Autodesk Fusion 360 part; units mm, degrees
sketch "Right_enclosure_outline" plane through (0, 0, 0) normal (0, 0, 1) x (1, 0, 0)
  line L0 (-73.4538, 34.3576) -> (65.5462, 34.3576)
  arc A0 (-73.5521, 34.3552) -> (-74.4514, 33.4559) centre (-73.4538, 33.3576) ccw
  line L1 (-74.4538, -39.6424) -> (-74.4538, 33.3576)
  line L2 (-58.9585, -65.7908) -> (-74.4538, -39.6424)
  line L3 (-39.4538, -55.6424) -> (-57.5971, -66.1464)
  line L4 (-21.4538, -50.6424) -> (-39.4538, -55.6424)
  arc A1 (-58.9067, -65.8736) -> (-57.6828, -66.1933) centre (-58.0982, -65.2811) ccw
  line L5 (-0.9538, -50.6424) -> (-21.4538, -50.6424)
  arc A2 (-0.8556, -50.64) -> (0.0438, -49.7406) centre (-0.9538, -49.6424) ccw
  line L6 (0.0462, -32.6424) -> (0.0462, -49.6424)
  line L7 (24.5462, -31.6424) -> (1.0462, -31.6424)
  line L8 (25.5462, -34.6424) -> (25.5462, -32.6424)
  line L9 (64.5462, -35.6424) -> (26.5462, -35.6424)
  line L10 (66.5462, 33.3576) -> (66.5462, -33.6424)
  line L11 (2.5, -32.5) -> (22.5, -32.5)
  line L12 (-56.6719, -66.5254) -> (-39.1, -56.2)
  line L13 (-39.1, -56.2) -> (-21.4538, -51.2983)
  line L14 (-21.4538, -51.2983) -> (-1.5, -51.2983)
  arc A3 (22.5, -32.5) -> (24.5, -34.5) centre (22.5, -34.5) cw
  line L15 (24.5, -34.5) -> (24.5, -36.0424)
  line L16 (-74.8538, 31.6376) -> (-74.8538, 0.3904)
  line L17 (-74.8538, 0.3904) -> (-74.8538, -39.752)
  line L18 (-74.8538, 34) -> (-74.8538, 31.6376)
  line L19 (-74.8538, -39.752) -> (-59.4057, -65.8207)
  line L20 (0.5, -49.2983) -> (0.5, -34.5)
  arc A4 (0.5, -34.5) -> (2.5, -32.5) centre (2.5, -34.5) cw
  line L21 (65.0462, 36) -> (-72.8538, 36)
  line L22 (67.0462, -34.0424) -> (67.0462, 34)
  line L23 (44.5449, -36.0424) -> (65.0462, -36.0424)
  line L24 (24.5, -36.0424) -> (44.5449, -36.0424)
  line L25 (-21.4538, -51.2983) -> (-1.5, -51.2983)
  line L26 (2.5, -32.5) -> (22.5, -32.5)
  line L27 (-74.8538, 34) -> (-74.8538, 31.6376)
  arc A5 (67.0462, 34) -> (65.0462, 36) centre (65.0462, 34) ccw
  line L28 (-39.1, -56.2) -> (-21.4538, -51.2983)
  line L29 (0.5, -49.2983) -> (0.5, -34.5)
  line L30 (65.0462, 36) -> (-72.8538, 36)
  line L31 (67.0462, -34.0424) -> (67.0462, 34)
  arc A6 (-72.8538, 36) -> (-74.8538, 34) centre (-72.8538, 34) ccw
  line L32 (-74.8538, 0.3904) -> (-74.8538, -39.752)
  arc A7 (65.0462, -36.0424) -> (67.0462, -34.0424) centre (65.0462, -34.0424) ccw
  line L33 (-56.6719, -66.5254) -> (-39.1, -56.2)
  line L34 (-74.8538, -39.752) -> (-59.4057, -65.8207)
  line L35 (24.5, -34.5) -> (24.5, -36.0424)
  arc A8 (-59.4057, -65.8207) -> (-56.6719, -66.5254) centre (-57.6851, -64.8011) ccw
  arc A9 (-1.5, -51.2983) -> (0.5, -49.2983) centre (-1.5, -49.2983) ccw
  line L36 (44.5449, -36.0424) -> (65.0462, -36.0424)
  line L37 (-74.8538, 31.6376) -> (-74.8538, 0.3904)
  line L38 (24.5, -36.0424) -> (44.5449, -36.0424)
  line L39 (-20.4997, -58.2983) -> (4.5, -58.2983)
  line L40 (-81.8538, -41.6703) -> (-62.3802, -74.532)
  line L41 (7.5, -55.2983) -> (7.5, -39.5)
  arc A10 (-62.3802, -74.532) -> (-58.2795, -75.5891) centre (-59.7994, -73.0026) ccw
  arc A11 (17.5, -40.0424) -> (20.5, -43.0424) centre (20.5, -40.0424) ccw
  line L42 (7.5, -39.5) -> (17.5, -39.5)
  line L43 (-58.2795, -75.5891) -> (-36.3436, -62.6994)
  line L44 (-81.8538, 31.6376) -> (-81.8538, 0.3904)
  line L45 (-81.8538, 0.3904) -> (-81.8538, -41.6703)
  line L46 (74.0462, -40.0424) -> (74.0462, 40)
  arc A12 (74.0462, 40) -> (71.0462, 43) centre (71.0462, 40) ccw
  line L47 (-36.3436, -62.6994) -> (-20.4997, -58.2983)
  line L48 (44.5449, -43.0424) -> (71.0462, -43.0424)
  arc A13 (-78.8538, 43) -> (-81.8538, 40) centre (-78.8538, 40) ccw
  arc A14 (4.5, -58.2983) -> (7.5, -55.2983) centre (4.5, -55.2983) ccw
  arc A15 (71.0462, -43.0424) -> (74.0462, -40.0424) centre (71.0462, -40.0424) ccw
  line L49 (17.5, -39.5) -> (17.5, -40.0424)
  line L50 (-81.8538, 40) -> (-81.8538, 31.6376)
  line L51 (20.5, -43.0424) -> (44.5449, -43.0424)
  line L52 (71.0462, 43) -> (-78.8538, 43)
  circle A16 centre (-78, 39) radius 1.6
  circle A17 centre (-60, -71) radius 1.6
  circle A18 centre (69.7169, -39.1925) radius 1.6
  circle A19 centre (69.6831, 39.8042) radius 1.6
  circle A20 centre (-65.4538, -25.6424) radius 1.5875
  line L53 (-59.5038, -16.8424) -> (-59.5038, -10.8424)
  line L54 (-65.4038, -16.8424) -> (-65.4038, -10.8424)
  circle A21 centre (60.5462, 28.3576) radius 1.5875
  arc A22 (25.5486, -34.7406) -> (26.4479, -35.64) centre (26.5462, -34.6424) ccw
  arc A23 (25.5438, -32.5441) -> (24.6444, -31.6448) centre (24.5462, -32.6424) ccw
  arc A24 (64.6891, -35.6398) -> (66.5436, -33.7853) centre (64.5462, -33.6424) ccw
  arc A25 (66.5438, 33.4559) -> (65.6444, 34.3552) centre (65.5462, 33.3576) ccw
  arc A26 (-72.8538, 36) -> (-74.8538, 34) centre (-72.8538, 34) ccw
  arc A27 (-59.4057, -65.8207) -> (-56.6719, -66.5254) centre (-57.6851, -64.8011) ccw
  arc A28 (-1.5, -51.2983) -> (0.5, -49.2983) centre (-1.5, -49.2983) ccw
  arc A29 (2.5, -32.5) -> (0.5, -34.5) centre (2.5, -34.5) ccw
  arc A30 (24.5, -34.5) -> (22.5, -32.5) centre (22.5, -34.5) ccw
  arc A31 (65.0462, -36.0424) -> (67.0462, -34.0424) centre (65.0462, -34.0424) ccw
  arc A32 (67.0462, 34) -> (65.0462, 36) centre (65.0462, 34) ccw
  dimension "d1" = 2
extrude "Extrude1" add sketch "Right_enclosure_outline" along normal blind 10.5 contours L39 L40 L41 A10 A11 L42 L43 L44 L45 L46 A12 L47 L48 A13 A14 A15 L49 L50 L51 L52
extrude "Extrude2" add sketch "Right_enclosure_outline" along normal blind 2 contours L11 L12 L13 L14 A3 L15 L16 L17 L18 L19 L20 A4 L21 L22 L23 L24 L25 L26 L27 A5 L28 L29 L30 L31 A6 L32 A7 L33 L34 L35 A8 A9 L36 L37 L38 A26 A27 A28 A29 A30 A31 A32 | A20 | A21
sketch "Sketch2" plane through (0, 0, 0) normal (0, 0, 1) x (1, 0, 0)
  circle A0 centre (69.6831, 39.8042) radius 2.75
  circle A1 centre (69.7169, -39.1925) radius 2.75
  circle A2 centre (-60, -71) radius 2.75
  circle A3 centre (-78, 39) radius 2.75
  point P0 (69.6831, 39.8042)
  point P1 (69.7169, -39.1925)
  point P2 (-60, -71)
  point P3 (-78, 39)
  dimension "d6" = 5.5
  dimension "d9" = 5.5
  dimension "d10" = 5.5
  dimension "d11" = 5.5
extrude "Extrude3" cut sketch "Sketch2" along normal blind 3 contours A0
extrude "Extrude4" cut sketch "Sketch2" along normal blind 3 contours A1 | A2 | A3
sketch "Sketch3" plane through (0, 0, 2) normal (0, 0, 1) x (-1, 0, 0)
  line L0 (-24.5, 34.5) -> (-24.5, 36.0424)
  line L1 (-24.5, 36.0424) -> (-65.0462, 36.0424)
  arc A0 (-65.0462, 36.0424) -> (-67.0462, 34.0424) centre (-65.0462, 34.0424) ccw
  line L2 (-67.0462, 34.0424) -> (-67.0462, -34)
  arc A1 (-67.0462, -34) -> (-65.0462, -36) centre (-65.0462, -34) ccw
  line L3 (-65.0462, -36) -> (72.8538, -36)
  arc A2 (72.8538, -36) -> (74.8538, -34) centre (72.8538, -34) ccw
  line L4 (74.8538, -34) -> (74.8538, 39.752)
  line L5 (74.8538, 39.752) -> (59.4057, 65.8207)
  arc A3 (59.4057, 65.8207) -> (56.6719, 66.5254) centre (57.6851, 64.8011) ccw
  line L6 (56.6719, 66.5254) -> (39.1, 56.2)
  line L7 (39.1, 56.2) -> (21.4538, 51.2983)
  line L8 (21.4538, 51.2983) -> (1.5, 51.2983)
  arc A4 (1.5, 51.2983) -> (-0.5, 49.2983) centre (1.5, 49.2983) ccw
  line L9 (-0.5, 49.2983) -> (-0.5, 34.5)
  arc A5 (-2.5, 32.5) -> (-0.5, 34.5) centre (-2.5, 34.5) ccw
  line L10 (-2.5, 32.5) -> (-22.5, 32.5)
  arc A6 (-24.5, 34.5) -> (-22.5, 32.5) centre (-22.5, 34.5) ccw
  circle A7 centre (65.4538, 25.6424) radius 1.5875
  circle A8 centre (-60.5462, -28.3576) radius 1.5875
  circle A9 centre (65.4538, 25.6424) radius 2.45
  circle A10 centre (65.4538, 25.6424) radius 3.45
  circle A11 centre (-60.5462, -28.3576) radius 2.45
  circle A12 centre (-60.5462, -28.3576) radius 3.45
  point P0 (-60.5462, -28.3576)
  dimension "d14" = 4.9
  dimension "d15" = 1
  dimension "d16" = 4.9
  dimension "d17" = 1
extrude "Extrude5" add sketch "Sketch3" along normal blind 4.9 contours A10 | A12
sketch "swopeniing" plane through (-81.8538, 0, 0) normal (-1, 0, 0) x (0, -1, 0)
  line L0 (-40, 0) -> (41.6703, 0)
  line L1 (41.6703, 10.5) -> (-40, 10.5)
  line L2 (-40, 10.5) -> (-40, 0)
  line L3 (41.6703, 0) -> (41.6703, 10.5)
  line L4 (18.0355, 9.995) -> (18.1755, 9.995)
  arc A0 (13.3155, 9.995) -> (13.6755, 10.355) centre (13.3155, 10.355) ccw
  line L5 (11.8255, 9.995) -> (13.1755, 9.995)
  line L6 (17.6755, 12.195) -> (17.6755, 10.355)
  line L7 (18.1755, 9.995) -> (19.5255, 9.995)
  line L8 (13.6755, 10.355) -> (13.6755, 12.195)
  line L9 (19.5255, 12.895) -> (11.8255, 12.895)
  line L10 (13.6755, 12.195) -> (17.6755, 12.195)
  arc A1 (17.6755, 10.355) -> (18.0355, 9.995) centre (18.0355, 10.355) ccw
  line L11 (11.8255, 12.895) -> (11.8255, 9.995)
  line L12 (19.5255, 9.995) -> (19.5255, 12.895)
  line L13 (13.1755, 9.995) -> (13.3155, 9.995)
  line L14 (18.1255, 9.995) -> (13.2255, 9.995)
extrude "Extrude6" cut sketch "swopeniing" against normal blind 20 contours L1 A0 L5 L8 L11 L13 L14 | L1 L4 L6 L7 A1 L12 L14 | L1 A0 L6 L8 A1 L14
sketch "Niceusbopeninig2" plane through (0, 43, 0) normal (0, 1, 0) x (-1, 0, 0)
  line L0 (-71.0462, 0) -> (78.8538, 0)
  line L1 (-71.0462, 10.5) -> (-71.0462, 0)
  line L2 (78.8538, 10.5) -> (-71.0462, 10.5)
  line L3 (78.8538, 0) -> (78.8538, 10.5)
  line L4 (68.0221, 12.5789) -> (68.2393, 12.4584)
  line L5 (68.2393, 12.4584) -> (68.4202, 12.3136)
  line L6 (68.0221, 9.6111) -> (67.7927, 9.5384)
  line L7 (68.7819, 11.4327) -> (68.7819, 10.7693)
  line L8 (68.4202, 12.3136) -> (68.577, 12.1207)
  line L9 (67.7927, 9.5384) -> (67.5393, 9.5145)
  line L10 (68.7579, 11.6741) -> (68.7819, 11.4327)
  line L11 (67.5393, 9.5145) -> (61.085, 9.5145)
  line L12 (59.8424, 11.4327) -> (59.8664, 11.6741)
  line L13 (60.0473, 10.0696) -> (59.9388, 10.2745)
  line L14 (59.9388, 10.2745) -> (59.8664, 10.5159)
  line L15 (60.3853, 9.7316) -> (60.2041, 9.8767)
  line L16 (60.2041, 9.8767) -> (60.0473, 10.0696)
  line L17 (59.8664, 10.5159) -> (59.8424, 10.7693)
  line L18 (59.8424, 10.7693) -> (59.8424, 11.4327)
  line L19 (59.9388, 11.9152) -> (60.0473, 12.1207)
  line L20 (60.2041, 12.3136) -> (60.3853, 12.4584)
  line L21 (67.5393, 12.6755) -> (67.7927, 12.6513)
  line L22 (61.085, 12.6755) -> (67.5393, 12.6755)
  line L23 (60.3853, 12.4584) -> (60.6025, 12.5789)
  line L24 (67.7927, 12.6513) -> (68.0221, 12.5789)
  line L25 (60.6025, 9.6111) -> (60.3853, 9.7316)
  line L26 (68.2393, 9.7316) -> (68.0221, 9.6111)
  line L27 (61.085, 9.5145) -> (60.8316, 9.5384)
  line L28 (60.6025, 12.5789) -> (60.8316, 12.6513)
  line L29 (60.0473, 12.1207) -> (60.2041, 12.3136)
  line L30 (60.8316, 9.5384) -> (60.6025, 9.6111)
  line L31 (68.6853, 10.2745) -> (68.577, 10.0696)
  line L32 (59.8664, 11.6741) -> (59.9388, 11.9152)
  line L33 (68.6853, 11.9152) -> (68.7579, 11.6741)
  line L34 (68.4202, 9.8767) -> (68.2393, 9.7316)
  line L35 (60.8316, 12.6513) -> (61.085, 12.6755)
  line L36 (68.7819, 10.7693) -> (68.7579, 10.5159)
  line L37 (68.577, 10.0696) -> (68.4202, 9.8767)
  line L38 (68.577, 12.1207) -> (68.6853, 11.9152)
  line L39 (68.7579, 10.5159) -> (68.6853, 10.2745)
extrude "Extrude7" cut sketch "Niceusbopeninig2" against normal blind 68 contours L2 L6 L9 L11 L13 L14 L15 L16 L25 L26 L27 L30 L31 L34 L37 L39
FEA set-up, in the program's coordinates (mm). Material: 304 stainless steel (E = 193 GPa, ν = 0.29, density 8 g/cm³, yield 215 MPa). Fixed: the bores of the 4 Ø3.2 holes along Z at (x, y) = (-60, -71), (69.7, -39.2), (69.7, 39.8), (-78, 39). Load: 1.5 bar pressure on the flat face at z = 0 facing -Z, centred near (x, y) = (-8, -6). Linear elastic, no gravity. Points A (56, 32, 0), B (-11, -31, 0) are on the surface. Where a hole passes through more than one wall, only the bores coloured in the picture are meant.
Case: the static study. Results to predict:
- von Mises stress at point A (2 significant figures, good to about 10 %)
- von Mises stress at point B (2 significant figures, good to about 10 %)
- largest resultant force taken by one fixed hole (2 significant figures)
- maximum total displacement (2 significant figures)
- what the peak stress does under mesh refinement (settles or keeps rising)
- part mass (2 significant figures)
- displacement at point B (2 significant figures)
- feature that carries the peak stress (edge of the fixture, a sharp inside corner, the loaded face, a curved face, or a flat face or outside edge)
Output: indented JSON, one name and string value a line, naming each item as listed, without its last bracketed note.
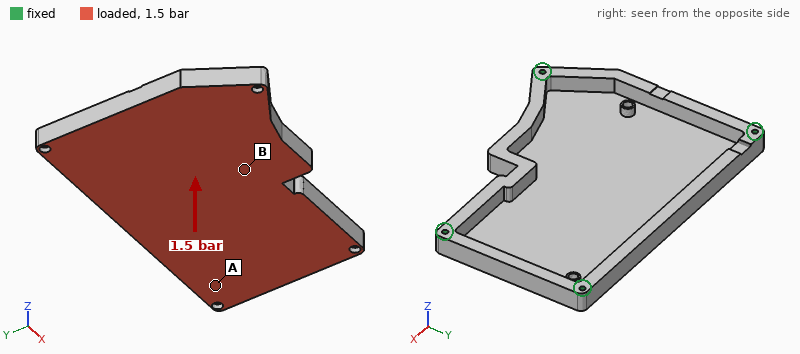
{
  "von Mises stress at point A": "17 MPa",
  "von Mises stress at point B": "33 MPa",
  "largest resultant force taken by one fixed hole": "1.3 kN",
  "maximum total displacement": "0.21 mm",
  "what the peak stress does under mesh refinement": "keeps rising",
  "part mass": "480 g",
  "displacement at point B": "0.13 mm",
  "feature that carries the peak stress": "edge of the fixture"
}
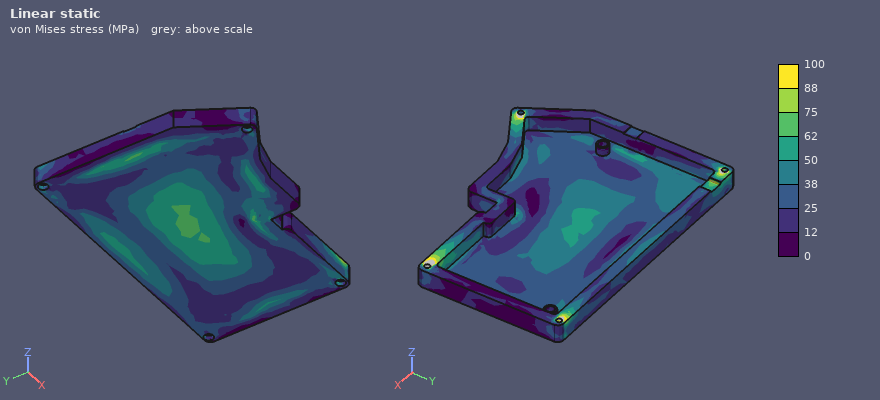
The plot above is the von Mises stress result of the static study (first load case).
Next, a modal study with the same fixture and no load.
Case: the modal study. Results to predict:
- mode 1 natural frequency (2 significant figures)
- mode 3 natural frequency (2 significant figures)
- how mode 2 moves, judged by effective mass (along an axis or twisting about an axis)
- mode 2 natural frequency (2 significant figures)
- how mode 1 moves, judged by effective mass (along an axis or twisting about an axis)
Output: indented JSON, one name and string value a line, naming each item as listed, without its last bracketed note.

{
  "mode 1 natural frequency": "1300 Hz",
  "mode 3 natural frequency": "2200 Hz",
  "how mode 2 moves, judged by effective mass": "twisting about X",
  "mode 2 natural frequency": "2000 Hz",
  "how mode 1 moves, judged by effective mass": "along Z"
}
